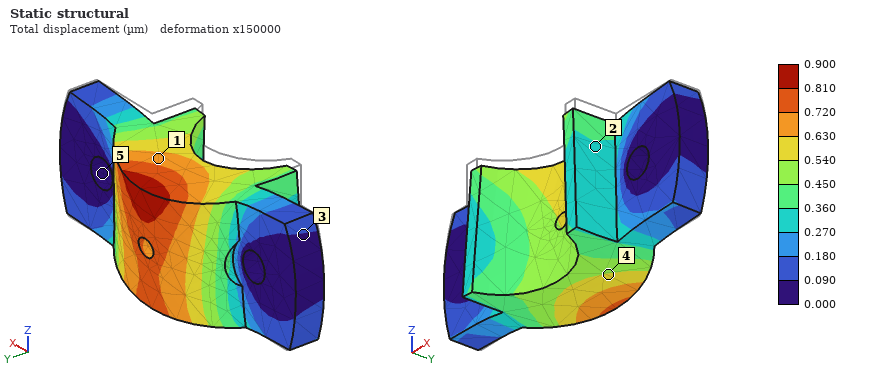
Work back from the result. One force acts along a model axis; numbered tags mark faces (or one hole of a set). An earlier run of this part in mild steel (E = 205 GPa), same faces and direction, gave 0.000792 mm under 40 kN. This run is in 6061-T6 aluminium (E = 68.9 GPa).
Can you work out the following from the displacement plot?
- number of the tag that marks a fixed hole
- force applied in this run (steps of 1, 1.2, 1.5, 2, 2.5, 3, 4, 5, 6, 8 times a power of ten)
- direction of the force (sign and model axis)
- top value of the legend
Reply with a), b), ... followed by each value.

a) 5
b) 15 kN
c) -Z
d) 0.900 µm
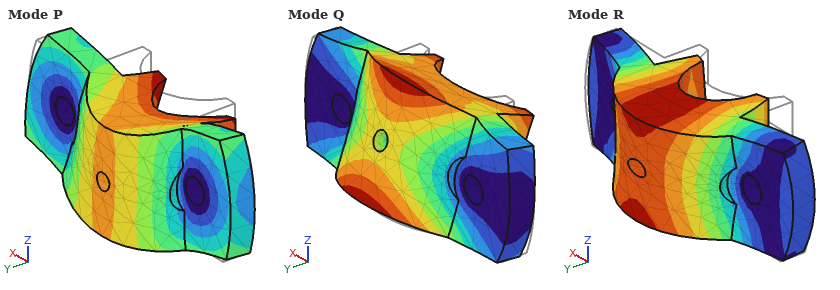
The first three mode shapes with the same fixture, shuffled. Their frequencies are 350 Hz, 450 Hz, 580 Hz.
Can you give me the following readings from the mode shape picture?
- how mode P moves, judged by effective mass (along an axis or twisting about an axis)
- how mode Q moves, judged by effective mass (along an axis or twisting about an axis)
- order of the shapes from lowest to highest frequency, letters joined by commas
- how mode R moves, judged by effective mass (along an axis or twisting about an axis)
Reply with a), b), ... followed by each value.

a) along Z
b) twisting about X
c) Q, R, P
d) along Y
